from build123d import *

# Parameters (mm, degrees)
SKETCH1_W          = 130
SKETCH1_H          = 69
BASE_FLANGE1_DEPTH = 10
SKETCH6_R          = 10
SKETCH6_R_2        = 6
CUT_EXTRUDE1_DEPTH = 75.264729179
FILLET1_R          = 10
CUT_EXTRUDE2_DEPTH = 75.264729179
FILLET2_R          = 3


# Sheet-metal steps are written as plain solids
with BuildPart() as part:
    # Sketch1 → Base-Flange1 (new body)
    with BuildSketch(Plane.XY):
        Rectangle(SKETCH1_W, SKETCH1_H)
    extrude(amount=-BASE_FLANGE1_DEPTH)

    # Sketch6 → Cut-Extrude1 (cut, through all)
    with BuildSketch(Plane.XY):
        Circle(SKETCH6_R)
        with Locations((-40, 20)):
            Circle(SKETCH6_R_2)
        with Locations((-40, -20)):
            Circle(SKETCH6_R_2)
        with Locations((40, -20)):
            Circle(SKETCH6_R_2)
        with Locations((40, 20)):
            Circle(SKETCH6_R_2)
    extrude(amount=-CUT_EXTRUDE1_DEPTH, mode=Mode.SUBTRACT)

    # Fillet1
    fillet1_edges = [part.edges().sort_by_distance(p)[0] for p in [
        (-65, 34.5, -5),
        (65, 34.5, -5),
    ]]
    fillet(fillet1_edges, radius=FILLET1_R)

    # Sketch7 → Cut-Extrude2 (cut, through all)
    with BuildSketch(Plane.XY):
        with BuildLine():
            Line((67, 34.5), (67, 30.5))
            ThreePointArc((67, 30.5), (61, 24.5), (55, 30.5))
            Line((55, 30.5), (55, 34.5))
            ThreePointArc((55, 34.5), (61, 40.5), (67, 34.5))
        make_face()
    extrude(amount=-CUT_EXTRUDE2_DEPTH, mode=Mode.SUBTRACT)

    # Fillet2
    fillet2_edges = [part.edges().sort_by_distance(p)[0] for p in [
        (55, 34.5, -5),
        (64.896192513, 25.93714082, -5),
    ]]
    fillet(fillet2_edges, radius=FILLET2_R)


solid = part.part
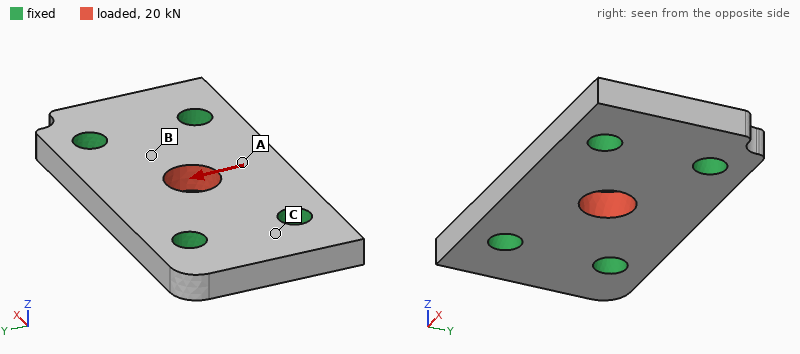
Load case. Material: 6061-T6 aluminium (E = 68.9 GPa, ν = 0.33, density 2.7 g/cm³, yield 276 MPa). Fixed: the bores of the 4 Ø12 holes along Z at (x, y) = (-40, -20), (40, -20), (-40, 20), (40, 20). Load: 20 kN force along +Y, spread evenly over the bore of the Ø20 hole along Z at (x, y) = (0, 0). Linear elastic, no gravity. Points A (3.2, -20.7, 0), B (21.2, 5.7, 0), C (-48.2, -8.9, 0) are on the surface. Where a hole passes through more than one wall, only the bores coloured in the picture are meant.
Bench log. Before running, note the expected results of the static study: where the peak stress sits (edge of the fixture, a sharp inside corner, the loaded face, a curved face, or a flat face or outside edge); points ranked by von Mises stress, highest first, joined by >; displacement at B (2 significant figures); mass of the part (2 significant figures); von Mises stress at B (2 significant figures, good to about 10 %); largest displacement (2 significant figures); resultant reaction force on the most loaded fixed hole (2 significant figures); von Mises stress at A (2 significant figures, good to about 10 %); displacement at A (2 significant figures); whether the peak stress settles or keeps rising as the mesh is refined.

edge of the fixture
B > A > C
12 µm
220 g
34 MPa
26 µm
6.1 kN
19 MPa
22 µm
keeps rising
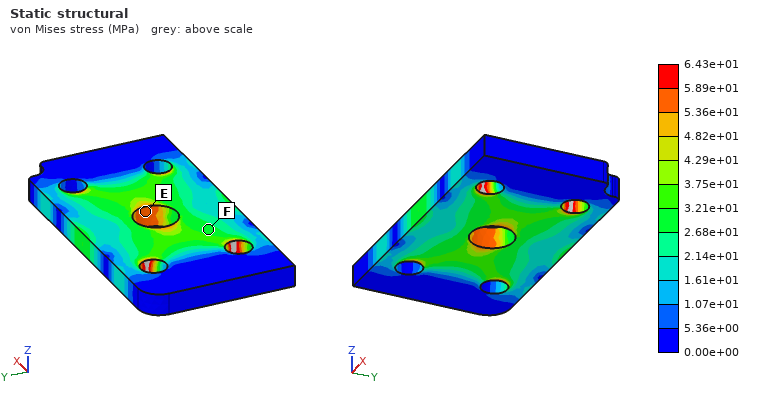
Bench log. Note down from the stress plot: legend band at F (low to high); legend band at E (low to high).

2.68e+01 to 3.21e+01 MPa
5.36e+01 to 5.89e+01 MPa
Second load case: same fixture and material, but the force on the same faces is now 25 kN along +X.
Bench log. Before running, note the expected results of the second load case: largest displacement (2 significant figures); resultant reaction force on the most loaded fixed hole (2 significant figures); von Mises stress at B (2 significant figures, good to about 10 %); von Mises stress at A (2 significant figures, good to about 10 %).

15 µm
6.5 kN
30 MPa
7.8 MPa
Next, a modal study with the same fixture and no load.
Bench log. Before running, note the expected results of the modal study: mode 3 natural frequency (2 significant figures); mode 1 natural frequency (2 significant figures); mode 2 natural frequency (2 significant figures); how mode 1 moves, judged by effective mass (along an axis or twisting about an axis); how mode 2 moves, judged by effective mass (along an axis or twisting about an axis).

14 kHz
8600 Hz
10 kHz
along Z
twisting about X
